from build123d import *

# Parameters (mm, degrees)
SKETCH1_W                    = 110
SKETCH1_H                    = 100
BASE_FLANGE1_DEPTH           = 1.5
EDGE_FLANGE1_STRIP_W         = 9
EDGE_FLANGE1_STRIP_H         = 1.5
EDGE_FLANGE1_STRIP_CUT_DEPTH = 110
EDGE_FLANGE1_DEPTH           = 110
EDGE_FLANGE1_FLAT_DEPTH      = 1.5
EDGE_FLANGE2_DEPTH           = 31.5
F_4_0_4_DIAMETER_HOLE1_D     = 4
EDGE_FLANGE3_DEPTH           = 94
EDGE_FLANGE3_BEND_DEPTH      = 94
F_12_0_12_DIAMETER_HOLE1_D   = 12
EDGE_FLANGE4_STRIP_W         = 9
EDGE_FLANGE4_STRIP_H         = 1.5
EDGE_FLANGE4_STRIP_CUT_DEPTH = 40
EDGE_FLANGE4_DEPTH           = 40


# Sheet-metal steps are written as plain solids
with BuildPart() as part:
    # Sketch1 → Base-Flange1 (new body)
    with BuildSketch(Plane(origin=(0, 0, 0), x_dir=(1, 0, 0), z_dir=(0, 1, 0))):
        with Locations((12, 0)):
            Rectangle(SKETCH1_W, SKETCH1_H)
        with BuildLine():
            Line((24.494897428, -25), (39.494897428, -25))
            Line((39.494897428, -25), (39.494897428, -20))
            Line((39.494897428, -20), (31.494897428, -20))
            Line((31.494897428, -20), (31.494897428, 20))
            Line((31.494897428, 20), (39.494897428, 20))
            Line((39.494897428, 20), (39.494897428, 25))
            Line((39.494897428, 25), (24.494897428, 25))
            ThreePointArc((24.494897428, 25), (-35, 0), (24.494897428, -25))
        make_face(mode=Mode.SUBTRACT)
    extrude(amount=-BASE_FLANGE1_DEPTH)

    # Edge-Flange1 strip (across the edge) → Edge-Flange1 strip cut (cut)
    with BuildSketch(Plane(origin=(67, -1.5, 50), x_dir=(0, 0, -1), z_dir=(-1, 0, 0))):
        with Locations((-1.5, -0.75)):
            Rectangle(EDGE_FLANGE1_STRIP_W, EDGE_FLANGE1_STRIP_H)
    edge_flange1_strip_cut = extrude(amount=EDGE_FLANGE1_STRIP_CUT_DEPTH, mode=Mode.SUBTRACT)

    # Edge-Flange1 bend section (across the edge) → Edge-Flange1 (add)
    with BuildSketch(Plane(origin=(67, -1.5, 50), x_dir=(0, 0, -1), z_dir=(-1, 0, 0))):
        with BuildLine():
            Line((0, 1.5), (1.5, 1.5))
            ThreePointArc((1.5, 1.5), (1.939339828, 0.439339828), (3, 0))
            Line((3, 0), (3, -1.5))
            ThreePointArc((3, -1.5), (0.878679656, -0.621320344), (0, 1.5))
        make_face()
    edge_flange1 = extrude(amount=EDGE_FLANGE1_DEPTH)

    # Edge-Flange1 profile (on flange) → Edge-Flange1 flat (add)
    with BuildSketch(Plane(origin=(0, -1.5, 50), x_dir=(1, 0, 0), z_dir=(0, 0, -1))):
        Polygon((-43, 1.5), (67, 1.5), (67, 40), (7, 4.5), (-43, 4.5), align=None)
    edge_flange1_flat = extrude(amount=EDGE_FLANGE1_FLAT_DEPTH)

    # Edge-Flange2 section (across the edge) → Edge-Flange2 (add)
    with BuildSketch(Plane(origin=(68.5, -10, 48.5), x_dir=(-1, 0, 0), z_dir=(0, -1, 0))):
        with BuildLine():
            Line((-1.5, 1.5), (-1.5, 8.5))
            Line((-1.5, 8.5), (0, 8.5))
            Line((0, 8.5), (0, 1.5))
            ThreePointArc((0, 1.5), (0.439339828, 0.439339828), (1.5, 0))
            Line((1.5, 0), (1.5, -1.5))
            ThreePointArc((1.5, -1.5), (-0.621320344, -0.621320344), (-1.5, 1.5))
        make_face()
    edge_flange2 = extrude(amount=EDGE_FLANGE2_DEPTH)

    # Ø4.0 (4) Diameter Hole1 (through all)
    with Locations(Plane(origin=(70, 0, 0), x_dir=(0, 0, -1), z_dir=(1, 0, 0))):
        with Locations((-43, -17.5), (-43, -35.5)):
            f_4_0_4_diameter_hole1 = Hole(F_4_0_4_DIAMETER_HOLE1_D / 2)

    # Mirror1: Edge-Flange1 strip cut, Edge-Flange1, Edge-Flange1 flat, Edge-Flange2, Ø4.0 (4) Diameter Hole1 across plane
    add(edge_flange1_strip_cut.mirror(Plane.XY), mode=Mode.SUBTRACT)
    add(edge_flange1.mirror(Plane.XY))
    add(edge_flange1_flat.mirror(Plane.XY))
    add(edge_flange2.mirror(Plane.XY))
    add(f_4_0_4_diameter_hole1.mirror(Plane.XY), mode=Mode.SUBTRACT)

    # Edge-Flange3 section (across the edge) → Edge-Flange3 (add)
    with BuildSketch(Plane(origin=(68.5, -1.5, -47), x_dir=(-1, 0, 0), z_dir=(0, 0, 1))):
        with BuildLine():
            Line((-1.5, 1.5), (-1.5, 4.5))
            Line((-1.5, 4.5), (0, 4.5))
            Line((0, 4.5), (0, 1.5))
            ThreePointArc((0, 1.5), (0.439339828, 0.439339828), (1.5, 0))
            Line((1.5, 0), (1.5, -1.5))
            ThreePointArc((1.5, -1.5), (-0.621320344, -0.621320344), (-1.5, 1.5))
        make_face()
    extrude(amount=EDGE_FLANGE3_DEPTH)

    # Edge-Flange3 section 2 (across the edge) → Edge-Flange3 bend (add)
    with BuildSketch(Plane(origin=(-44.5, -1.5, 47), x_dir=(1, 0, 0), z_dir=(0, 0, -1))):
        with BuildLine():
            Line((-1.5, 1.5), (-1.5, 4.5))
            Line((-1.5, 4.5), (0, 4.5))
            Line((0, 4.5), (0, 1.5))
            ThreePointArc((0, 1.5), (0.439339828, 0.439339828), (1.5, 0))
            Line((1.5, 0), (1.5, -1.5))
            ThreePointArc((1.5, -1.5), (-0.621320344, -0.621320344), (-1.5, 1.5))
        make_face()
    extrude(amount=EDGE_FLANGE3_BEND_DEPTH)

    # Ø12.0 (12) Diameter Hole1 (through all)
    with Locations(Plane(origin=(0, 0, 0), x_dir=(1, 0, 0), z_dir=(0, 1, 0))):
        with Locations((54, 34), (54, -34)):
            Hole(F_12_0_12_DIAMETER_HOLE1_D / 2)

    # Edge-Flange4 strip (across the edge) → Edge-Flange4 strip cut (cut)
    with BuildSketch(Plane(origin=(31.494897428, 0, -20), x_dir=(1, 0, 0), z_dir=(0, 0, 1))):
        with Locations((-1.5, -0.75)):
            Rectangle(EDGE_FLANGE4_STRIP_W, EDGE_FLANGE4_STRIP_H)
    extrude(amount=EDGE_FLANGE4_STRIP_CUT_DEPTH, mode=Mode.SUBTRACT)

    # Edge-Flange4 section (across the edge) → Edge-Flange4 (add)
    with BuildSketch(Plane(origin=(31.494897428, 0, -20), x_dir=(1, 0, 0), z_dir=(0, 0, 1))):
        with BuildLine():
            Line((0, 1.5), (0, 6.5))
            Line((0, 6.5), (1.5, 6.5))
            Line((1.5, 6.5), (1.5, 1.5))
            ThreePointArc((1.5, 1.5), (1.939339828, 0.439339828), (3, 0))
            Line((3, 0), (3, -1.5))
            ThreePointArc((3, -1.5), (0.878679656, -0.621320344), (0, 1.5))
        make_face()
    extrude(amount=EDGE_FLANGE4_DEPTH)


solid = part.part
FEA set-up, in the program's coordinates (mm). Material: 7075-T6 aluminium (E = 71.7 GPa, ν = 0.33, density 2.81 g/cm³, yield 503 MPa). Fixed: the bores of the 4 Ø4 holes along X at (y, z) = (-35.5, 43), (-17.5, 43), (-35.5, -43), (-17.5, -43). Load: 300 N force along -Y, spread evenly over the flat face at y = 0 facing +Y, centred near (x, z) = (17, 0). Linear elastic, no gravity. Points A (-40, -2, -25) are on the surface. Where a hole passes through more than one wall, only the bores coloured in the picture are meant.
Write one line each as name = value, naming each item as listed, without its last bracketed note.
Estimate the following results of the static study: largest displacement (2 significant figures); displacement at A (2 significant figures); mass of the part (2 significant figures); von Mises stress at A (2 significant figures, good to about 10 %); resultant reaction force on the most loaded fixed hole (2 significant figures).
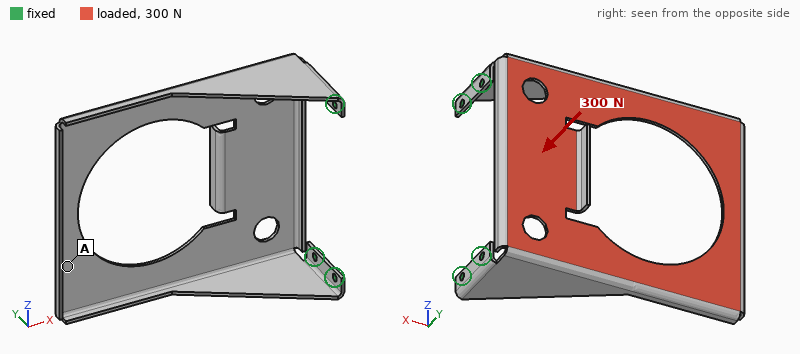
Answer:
largest displacement = 1.6 mm
displacement at A = 1.5 mm
mass of the part = 50 g
von Mises stress at A = 21 MPa
resultant reaction force on the most loaded fixed hole = 420 N
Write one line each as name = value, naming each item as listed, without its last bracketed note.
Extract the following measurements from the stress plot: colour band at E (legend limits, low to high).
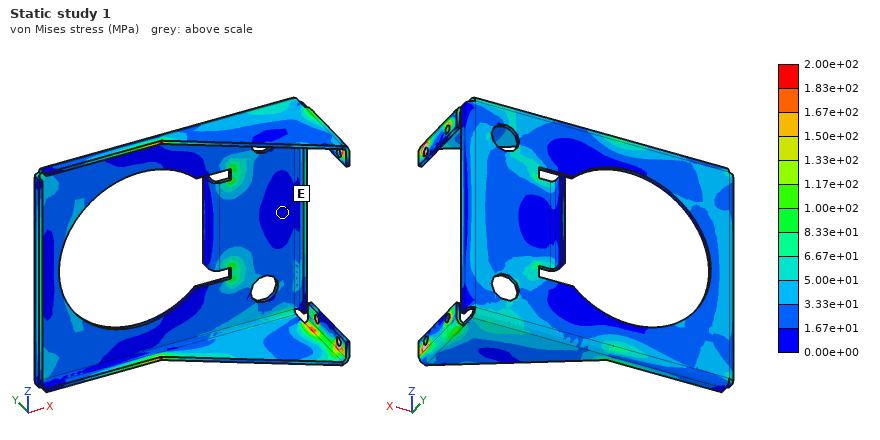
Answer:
colour band at E = 0.00e+00 to 1.67e+01 MPa
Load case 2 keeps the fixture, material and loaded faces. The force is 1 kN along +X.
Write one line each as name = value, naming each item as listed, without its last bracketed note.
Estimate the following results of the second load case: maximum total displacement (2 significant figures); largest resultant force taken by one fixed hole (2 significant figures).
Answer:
maximum total displacement = 1.2 mm
largest resultant force taken by one fixed hole = 930 N
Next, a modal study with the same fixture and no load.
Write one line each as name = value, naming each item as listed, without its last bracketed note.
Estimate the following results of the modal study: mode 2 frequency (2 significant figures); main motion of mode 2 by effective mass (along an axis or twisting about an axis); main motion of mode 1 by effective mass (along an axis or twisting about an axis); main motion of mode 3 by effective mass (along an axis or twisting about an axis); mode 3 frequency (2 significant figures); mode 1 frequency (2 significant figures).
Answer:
mode 2 frequency = 520 Hz
main motion of mode 2 by effective mass = along Z
main motion of mode 1 by effective mass = along Y
main motion of mode 3 by effective mass = along Y
mode 3 frequency = 790 Hz
mode 1 frequency = 410 Hz
